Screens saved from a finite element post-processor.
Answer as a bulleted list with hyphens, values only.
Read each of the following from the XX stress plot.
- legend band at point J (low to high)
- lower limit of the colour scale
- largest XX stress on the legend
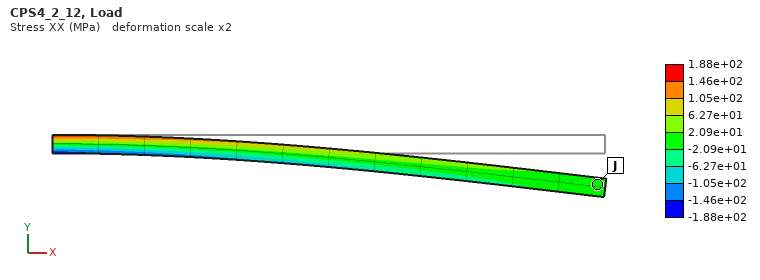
- -2.09e+01 to 2.09e+01 MPa
- -1.88e+02 MPa
- 1.88e+02 MPa
